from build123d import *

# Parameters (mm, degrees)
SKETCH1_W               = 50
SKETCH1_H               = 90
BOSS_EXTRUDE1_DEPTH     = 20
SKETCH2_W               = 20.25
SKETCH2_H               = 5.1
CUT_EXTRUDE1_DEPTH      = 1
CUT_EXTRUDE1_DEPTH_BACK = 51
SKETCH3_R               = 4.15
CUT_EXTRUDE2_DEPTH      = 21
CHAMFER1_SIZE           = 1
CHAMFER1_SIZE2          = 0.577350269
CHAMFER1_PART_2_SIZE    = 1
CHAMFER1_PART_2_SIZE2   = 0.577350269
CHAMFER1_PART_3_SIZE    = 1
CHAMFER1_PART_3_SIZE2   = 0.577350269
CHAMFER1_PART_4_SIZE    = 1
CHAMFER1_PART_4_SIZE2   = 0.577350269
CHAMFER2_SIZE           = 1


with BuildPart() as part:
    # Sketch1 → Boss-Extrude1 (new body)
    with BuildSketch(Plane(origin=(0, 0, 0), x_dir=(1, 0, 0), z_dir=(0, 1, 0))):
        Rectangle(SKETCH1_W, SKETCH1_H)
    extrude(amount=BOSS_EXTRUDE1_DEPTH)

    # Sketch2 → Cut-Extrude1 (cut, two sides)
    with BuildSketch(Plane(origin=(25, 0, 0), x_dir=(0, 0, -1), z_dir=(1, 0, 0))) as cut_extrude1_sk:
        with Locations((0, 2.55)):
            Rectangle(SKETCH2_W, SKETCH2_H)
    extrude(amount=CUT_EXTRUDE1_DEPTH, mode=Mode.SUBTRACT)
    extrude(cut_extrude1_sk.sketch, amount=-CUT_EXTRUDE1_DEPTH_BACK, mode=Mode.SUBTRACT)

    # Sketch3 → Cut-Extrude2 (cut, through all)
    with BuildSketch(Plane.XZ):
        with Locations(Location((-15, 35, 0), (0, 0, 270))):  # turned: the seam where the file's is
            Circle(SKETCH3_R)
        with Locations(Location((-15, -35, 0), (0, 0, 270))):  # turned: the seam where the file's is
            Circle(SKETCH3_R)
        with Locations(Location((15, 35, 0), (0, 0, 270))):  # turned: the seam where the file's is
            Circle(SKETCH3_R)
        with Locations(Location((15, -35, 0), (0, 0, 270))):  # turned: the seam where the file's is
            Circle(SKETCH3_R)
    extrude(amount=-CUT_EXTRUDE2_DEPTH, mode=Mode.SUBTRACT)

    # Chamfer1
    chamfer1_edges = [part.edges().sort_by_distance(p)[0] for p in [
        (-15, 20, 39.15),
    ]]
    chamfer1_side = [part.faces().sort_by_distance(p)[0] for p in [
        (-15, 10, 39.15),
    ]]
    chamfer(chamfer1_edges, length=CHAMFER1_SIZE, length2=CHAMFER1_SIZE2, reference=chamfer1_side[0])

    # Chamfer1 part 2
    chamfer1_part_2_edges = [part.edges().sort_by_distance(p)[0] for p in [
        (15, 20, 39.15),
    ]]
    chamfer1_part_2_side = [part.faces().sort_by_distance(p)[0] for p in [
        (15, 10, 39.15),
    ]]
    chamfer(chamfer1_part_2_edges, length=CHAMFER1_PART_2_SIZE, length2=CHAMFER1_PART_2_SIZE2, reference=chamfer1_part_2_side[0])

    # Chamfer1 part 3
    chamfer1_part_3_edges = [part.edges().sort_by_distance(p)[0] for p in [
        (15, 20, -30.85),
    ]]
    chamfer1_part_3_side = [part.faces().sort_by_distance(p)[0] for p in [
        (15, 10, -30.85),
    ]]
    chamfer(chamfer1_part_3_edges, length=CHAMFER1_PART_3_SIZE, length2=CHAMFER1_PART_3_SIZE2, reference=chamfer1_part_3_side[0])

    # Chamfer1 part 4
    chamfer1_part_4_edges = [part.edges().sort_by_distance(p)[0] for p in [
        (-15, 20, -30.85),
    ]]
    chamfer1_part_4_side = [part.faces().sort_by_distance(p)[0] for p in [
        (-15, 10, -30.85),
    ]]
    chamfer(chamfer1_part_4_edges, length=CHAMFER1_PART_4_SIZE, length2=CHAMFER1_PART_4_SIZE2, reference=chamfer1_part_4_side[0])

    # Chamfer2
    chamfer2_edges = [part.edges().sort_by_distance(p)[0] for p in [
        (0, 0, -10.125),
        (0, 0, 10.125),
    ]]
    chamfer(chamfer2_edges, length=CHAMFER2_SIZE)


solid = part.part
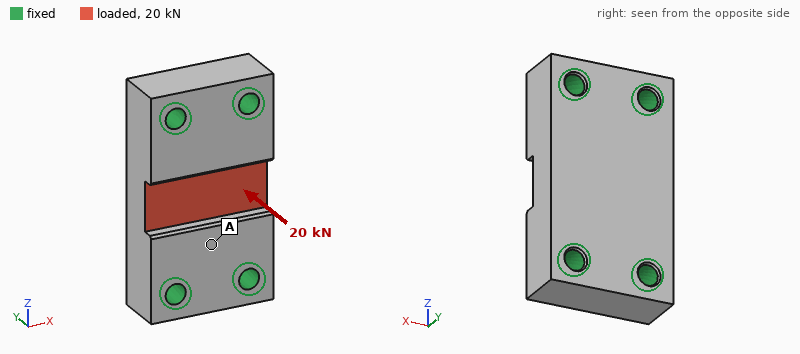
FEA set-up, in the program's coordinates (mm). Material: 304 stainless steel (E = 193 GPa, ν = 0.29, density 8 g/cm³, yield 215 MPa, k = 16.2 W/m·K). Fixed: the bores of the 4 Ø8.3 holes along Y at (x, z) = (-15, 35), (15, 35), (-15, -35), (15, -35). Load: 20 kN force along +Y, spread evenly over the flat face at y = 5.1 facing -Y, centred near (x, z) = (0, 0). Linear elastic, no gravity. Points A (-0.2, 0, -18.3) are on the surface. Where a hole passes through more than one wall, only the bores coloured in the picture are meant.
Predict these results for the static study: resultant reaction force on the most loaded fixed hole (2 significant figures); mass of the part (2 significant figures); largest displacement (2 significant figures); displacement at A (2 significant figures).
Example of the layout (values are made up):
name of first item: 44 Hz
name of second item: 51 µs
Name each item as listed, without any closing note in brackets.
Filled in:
resultant reaction force on the most loaded fixed hole: 5.3 kN
mass of the part: 640 g
largest displacement: 13 µm
displacement at A: 6.7 µm
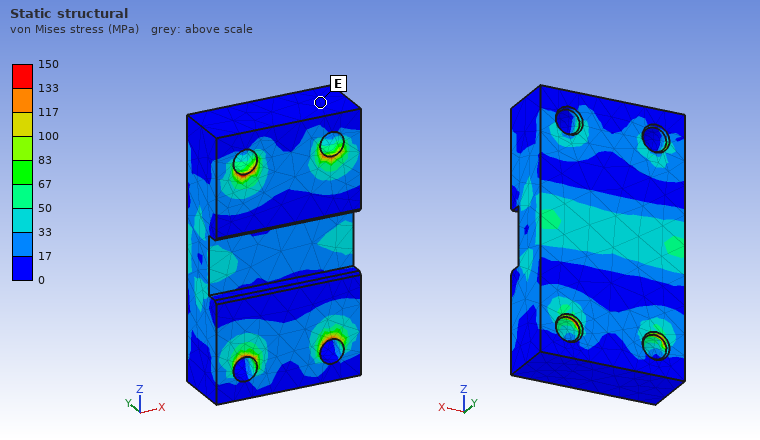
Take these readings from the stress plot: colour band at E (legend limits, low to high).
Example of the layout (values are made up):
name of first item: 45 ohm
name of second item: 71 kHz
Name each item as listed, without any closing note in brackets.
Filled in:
colour band at E: 0 to 17 MPa
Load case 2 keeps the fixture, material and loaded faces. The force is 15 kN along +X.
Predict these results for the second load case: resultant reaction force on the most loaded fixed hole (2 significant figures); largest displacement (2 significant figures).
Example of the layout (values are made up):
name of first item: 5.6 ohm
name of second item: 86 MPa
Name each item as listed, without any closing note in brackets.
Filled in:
resultant reaction force on the most loaded fixed hole: 5.0 kN
largest displacement: 7.8 µm
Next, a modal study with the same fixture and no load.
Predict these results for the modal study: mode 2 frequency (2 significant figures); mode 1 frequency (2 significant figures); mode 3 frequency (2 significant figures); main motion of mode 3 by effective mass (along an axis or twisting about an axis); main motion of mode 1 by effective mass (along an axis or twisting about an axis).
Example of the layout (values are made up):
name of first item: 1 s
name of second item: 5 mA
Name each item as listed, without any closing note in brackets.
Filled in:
mode 2 frequency: 19 kHz
mode 1 frequency: 15 kHz
mode 3 frequency: 21 kHz
main motion of mode 3 by effective mass: along X
main motion of mode 1 by effective mass: along Y
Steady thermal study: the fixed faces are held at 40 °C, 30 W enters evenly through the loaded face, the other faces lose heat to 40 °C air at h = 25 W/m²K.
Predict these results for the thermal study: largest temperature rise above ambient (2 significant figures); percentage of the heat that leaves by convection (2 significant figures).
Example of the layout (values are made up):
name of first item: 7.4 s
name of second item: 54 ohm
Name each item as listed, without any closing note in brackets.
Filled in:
largest temperature rise above ambient: 36 K
percentage of the heat that leaves by convection: 9.8 %
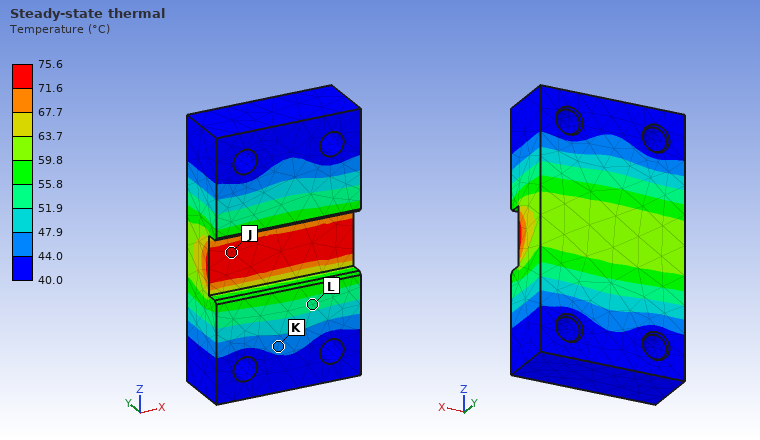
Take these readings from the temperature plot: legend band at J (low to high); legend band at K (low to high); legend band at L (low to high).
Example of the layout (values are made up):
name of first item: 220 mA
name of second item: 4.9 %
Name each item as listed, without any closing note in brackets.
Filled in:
legend band at J: 71.6 to 75.6 °C
legend band at K: 44.0 to 47.9 °C
legend band at L: 51.9 to 55.8 °C
